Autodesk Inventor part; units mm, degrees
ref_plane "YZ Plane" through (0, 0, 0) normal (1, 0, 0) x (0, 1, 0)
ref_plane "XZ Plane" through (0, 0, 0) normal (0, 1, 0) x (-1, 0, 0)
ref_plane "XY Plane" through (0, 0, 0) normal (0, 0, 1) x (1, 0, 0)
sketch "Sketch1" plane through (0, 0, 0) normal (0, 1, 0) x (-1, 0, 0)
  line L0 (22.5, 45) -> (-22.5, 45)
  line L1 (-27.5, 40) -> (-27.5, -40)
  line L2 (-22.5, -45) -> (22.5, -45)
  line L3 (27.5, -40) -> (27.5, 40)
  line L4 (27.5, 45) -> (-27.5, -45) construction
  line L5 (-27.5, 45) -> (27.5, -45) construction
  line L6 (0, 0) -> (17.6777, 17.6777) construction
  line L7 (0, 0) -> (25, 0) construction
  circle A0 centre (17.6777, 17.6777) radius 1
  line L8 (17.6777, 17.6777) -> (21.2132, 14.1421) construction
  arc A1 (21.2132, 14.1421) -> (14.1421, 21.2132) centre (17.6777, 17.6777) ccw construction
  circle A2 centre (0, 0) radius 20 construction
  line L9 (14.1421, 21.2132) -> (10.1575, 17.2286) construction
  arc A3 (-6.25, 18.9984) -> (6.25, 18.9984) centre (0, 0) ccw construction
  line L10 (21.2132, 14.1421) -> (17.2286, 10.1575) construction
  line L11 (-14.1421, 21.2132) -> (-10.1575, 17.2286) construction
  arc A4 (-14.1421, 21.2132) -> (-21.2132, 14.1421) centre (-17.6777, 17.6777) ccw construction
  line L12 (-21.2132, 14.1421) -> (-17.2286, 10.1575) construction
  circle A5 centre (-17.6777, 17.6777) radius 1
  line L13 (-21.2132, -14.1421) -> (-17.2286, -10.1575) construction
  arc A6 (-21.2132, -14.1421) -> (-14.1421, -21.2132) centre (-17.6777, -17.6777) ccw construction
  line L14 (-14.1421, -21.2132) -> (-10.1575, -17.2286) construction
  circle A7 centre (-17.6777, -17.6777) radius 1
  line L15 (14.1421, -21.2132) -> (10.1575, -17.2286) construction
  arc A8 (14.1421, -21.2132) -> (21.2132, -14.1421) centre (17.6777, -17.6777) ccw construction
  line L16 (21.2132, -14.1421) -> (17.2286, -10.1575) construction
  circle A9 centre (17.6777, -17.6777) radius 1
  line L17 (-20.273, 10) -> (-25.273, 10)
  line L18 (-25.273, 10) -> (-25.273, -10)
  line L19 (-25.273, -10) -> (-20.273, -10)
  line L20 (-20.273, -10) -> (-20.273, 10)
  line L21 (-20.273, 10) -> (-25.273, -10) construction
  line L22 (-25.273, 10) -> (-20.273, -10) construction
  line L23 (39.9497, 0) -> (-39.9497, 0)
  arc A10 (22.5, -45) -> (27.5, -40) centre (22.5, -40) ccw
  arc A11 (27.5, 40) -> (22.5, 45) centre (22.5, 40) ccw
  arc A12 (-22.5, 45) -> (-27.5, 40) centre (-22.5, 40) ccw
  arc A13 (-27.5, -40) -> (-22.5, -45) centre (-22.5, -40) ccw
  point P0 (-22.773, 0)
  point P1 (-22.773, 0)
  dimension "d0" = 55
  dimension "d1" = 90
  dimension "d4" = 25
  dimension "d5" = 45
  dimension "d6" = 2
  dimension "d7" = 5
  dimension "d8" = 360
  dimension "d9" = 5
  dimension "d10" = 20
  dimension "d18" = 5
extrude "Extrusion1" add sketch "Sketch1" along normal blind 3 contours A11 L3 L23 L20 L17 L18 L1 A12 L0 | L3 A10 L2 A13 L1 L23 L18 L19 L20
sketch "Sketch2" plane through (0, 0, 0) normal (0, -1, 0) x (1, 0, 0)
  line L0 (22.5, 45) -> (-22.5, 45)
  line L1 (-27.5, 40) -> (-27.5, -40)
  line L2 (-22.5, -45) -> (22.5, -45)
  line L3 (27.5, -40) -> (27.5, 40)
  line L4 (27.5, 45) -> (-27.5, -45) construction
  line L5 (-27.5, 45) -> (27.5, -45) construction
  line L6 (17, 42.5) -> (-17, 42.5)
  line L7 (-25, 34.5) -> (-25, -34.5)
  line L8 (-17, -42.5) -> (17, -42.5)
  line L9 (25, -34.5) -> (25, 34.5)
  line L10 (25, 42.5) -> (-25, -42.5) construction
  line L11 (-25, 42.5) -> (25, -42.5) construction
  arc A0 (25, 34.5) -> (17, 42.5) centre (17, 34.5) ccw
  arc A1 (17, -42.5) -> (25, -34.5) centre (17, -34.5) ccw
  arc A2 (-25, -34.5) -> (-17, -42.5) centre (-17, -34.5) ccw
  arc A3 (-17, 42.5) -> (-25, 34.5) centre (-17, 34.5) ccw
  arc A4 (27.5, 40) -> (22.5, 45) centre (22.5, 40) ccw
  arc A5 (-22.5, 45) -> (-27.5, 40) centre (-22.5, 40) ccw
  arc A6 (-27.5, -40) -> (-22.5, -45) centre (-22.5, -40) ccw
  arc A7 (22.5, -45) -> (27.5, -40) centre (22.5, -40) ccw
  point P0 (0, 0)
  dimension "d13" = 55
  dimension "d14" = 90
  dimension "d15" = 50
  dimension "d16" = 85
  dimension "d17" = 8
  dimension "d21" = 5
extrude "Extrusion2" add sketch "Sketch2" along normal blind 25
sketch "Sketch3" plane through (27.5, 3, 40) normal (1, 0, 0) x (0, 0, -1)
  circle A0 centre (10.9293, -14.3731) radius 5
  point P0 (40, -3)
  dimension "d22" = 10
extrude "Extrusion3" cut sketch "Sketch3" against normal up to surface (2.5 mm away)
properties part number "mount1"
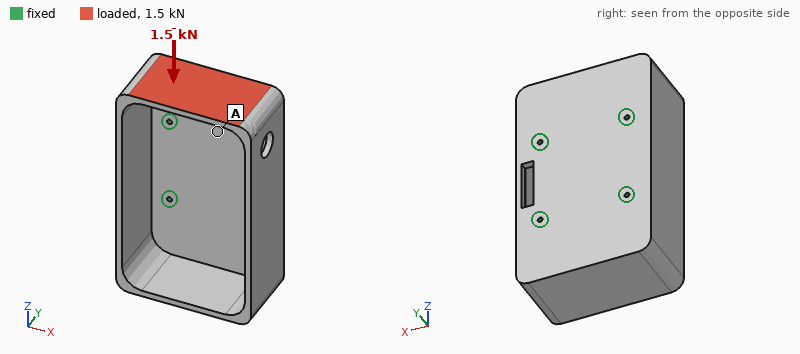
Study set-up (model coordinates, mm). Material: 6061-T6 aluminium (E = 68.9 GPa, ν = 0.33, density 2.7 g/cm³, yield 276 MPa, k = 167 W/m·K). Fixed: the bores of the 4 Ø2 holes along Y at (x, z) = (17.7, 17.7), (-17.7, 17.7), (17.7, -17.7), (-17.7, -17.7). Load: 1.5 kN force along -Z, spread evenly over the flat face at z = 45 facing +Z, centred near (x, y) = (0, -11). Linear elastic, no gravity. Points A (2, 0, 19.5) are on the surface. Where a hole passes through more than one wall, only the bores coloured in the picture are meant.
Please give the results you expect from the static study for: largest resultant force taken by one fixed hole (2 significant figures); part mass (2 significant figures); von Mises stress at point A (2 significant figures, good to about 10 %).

530 N
88 g
13 MPa
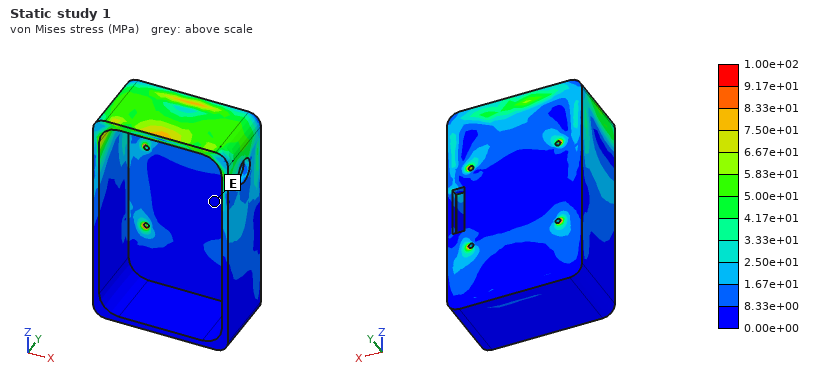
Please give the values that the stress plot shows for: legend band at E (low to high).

0.00e+00 to 8.33e+00 MPa
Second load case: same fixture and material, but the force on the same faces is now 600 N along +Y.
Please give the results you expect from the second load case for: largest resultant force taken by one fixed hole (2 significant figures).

520 N
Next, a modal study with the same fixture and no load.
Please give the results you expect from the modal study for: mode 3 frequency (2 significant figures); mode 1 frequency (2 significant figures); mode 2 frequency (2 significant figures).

2800 Hz
2600 Hz
2800 Hz
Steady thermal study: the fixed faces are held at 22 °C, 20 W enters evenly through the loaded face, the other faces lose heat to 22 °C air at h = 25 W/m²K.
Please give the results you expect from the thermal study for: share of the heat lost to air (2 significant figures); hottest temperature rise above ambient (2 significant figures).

14 %
21 K
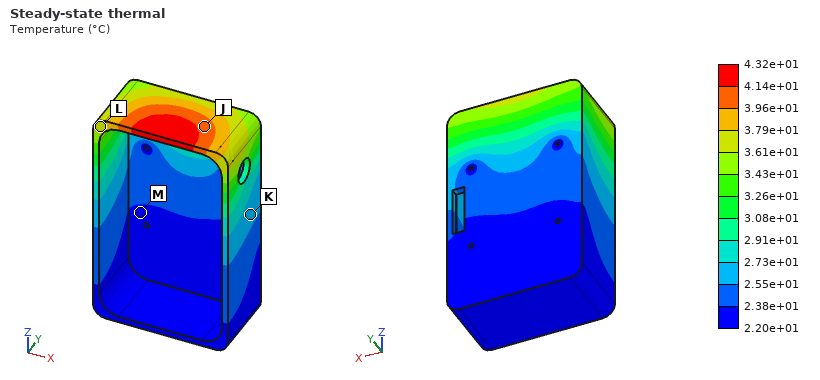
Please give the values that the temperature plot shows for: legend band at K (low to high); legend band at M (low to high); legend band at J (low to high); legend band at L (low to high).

2.55e+01 to 2.73e+01 °C
2.20e+01 to 2.38e+01 °C
3.96e+01 to 4.14e+01 °C
3.61e+01 to 3.79e+01 °C
